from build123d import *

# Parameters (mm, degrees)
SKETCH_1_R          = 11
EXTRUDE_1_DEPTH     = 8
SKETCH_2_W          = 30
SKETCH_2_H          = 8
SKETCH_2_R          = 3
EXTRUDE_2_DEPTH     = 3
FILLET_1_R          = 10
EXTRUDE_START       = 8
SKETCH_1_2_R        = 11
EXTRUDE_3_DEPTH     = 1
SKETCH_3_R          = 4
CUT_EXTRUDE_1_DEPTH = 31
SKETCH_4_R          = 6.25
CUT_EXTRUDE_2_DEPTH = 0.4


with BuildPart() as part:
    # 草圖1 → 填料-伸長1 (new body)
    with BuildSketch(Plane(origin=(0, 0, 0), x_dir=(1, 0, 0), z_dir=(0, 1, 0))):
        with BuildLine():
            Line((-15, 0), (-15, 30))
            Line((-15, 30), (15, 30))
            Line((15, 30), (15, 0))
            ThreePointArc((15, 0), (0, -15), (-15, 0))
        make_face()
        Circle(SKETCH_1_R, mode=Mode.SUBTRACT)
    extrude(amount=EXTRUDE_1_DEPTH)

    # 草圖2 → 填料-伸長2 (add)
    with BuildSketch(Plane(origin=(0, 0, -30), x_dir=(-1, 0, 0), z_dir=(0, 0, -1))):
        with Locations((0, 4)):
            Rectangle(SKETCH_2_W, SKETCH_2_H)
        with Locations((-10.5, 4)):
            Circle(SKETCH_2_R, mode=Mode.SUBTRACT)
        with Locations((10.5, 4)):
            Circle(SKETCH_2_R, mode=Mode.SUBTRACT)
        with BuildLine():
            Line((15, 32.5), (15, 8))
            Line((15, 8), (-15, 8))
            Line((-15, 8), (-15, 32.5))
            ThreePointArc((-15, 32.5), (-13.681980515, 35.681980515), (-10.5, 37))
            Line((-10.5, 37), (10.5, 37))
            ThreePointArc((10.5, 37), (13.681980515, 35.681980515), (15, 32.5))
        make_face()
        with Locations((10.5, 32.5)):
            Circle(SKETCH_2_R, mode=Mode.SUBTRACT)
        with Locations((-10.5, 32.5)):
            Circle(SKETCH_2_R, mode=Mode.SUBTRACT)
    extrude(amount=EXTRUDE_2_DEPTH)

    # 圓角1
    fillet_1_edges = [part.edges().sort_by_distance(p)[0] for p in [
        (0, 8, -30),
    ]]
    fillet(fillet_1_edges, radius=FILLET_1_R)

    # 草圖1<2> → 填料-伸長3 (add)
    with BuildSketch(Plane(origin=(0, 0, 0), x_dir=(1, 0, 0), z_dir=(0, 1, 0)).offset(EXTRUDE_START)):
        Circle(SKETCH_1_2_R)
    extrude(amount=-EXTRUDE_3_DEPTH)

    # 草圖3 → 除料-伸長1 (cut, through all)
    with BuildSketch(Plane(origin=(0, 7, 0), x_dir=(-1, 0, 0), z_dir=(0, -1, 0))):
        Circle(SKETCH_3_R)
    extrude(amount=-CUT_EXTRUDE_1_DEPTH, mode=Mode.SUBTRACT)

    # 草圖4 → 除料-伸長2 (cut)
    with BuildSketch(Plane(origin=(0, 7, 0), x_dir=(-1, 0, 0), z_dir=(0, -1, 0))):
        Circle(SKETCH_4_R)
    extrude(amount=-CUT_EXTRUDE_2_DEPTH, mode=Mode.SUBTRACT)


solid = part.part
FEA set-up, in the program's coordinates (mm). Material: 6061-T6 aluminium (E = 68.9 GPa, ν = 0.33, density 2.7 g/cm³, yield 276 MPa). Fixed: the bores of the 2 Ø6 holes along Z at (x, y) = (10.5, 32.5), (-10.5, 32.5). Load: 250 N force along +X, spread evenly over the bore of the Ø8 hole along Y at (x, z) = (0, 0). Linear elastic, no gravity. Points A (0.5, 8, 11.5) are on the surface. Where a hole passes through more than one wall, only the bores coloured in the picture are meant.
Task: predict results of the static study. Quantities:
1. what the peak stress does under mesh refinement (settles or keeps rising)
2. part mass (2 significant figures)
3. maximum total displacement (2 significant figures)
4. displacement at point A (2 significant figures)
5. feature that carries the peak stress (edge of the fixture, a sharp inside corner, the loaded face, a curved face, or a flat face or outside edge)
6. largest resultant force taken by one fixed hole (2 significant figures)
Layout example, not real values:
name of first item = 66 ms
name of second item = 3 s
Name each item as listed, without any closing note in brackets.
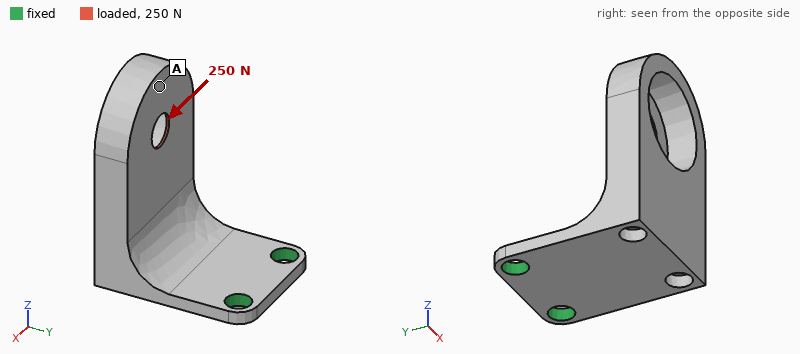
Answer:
what the peak stress does under mesh refinement = keeps rising
part mass = 29 g
maximum total displacement = 0.37 mm
displacement at point A = 0.34 mm
feature that carries the peak stress = edge of the fixture
largest resultant force taken by one fixed hole = 450 N
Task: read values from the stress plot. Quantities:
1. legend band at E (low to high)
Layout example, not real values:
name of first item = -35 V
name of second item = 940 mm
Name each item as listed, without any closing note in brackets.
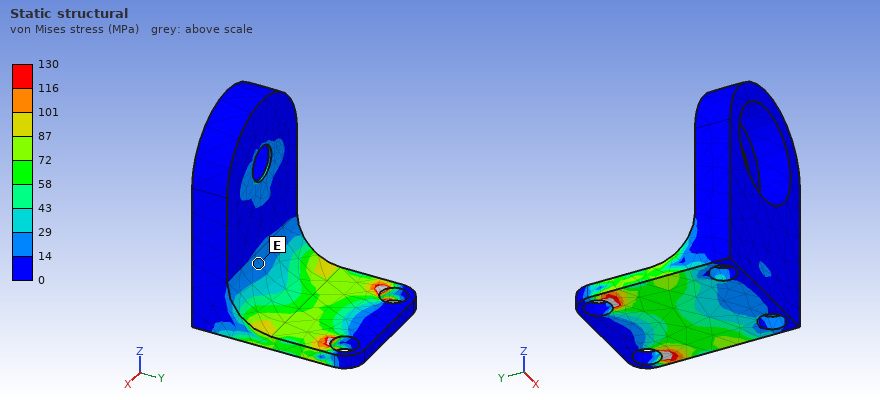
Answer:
legend band at E = 14 to 29 MPa
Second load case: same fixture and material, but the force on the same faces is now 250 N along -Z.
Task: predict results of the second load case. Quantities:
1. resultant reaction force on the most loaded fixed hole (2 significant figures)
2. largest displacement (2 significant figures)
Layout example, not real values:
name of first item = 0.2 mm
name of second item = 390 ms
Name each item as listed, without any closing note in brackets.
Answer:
resultant reaction force on the most loaded fixed hole = 130 N
largest displacement = 0.65 mm
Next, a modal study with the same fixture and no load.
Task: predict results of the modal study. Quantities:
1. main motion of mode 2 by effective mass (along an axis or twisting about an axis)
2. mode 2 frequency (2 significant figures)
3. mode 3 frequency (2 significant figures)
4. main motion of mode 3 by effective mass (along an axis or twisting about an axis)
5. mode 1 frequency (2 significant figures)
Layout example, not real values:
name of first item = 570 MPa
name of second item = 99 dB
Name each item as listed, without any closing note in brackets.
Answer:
main motion of mode 2 by effective mass = along X
mode 2 frequency = 1400 Hz
mode 3 frequency = 3500 Hz
main motion of mode 3 by effective mass = along Z
mode 1 frequency = 630 Hz
